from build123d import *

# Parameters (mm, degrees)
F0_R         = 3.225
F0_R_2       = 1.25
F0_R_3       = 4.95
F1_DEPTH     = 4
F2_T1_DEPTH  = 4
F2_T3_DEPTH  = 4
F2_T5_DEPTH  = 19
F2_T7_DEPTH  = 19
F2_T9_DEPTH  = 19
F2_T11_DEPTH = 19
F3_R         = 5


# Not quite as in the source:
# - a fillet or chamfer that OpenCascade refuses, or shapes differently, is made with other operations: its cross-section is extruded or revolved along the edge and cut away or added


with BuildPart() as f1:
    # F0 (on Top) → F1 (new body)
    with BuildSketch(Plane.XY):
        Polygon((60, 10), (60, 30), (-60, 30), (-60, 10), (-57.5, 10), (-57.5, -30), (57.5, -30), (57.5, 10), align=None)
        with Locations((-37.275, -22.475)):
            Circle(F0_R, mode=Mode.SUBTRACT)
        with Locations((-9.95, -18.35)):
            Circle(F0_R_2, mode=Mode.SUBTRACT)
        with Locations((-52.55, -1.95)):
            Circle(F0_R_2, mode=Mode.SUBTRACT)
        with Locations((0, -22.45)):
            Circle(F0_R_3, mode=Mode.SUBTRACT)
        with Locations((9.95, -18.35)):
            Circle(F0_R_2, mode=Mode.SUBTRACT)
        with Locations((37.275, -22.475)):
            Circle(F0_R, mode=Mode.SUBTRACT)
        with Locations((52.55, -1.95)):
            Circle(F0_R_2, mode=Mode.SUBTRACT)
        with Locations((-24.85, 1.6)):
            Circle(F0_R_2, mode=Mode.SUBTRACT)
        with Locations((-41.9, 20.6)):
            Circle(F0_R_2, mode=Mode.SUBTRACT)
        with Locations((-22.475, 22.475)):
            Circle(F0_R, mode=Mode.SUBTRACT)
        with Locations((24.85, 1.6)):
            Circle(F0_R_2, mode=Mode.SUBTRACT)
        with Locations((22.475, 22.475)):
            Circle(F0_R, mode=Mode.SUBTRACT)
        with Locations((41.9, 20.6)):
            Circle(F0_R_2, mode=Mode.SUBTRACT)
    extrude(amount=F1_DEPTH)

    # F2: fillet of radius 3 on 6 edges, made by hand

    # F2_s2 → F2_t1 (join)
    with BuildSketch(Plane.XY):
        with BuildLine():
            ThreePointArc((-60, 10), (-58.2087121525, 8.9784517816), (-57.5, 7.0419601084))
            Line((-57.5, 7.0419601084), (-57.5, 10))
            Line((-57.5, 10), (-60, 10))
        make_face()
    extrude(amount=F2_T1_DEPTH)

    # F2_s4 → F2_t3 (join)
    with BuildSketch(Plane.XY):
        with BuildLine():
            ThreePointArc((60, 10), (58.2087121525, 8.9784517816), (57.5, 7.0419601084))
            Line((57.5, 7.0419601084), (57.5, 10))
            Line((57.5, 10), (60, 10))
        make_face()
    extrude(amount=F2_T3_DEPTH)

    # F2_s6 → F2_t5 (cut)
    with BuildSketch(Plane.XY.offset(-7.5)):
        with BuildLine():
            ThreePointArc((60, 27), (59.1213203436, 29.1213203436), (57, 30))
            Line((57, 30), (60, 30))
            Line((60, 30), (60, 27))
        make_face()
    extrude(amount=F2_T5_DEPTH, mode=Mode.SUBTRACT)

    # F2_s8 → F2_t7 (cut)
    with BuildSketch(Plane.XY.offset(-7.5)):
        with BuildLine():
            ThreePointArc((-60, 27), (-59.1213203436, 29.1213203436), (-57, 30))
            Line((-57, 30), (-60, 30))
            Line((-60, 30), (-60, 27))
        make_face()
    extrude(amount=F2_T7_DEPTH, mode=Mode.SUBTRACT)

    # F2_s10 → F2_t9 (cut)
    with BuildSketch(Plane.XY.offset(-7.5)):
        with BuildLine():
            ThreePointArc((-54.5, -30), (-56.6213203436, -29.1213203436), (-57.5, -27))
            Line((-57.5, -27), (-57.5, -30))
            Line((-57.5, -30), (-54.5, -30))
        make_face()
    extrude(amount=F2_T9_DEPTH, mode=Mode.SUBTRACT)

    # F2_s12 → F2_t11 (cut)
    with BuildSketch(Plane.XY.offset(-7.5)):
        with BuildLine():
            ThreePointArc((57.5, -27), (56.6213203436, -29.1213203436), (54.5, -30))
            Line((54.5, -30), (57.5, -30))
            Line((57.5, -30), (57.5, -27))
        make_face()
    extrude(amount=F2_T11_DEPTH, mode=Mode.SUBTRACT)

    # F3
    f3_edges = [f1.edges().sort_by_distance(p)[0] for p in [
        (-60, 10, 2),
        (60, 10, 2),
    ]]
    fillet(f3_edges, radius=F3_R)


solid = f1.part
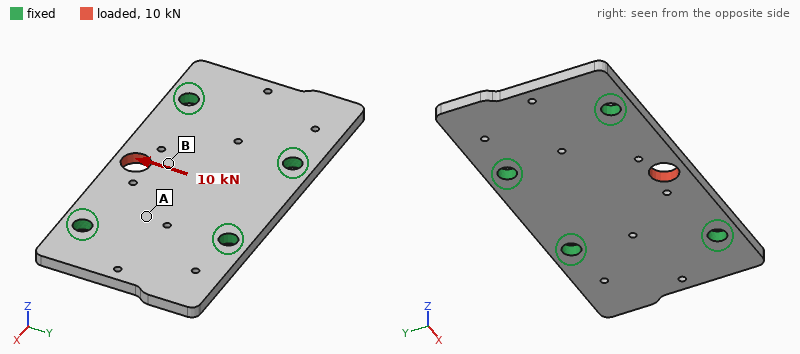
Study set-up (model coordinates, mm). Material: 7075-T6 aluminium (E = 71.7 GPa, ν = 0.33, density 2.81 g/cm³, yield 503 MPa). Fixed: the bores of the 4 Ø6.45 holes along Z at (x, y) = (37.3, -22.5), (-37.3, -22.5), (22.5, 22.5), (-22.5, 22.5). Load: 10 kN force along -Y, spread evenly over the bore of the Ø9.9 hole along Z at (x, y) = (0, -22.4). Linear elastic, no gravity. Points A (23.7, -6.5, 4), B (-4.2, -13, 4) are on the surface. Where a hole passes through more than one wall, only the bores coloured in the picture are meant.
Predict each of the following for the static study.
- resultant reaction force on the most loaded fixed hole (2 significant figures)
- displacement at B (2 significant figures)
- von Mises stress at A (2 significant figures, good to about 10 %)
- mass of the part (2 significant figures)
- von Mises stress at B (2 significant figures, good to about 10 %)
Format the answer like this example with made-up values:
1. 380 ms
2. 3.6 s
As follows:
1. 3.7 kN
2. 32 µm
3. 35 MPa
4. 76 g
5. 86 MPa
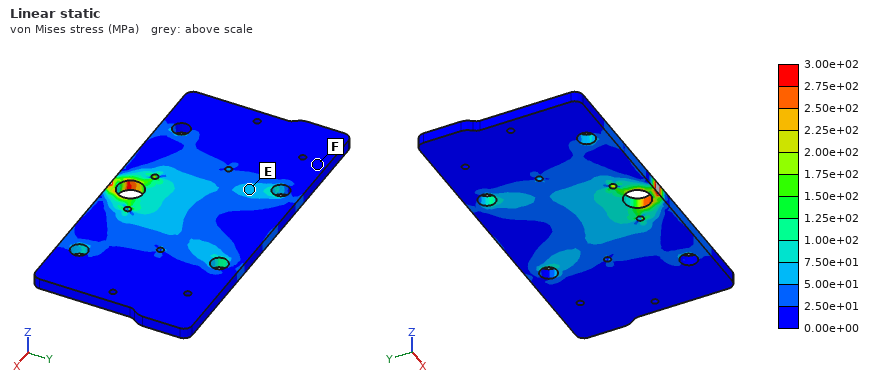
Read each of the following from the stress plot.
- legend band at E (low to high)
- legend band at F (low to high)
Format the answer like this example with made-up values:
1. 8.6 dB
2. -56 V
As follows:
1. 5.00e+01 to 7.50e+01 MPa
2. 0.00e+00 to 2.50e+01 MPa
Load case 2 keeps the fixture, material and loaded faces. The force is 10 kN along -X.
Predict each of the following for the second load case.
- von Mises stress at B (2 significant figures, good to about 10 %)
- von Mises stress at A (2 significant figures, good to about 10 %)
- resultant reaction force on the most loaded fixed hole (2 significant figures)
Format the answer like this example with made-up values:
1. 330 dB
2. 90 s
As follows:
1. 44 MPa
2. 16 MPa
3. 4.0 kN
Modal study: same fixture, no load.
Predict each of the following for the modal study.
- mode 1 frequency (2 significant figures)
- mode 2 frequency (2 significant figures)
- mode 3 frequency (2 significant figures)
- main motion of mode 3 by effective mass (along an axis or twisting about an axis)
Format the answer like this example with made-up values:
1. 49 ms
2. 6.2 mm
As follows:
1. 3300 Hz
2. 3300 Hz
3. 4600 Hz
4. along Z
